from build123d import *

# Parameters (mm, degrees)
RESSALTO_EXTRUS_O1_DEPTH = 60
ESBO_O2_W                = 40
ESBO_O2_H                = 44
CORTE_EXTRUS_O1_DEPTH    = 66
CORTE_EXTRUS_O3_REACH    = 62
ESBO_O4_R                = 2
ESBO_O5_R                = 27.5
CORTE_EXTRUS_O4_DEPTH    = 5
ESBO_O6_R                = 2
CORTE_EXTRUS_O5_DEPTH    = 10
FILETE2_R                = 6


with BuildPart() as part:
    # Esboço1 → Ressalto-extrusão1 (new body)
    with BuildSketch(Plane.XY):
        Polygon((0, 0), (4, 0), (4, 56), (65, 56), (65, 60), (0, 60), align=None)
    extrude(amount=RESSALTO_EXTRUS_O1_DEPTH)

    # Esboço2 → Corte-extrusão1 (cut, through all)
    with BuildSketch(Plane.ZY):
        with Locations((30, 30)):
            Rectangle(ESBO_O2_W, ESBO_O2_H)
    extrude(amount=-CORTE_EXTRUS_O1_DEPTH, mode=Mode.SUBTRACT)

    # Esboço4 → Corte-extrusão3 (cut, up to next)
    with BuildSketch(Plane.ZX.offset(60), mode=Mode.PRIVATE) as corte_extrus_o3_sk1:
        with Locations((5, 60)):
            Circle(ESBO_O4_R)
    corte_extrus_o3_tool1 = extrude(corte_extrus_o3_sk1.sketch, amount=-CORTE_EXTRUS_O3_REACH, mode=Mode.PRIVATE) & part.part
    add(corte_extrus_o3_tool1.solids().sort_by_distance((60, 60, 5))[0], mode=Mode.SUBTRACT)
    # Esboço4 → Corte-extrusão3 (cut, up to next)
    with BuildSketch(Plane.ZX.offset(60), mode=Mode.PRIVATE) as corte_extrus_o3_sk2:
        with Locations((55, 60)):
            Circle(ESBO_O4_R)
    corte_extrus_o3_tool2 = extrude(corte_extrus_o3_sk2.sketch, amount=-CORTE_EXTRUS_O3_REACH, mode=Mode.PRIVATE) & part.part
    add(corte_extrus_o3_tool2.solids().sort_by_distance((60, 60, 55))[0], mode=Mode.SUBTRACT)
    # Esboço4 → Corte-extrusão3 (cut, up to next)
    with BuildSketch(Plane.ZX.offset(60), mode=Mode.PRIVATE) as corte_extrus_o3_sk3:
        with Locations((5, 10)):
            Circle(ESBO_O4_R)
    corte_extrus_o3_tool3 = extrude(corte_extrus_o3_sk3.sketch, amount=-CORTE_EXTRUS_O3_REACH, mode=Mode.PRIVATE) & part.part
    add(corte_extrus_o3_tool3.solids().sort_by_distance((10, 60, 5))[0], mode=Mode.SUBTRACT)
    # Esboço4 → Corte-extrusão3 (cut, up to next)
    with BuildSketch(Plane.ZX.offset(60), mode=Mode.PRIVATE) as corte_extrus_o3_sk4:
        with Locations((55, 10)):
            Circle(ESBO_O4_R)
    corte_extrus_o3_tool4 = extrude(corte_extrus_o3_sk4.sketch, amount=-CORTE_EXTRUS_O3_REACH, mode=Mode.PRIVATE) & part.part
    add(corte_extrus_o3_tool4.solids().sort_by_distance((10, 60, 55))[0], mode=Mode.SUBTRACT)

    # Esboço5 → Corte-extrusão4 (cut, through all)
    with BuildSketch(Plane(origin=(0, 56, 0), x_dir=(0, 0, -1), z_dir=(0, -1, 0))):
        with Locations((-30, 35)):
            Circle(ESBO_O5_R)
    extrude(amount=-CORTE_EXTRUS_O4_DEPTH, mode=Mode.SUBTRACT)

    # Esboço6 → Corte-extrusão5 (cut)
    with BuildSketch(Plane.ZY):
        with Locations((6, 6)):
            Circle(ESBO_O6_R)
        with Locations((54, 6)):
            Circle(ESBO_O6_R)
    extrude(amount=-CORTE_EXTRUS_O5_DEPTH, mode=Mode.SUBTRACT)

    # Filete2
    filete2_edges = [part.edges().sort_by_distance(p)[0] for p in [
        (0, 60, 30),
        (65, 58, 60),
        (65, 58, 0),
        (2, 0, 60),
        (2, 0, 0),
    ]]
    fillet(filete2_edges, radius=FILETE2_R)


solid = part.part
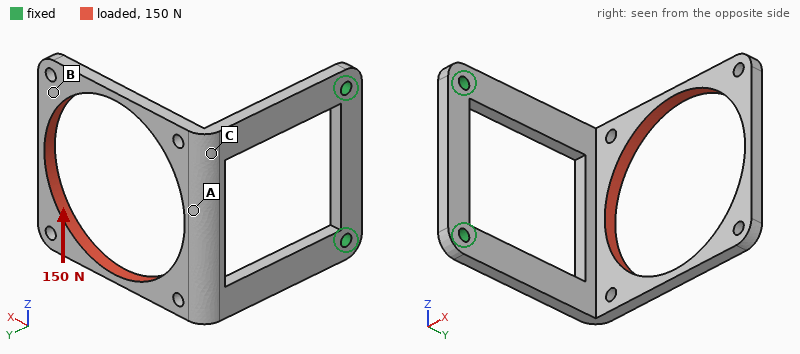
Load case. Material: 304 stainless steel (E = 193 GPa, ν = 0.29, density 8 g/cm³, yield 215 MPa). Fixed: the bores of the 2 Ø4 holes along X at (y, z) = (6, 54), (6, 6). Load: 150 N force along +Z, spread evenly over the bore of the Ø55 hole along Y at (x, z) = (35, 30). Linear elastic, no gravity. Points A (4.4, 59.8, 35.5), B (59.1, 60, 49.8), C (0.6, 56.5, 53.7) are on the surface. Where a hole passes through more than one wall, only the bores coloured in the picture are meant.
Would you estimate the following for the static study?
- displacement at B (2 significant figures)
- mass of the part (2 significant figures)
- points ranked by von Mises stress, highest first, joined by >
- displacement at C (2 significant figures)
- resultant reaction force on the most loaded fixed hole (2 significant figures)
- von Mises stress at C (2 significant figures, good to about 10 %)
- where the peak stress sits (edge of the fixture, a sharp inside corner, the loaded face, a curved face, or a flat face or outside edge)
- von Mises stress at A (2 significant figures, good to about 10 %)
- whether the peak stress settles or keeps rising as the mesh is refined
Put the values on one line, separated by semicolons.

0.31 mm; 93 g; C > A > B; 0.10 mm; 130 N; 53 MPa; edge of the fixture; 34 MPa; keeps rising
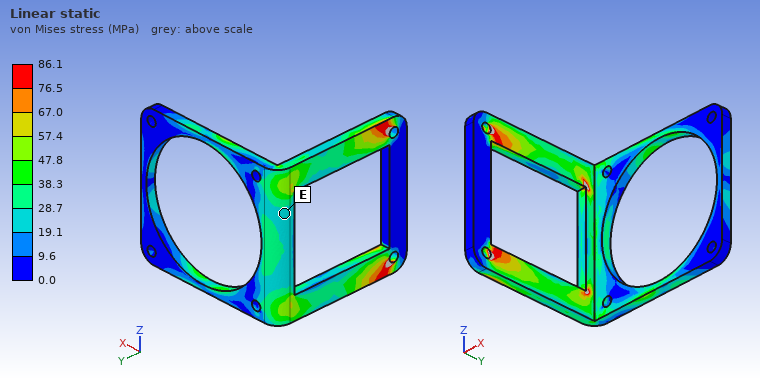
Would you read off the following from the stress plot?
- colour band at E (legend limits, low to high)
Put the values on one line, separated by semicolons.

19.1 to 28.7 MPa
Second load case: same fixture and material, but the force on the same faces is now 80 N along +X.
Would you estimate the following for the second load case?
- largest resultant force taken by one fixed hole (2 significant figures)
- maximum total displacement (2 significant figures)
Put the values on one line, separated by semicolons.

40 N; 0.37 mm
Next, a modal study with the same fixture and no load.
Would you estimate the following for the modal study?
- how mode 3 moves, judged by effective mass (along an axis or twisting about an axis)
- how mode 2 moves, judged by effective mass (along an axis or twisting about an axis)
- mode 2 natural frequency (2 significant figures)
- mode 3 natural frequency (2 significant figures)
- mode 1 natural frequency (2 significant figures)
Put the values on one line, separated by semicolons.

along X; along Z; 550 Hz; 730 Hz; 300 Hz
